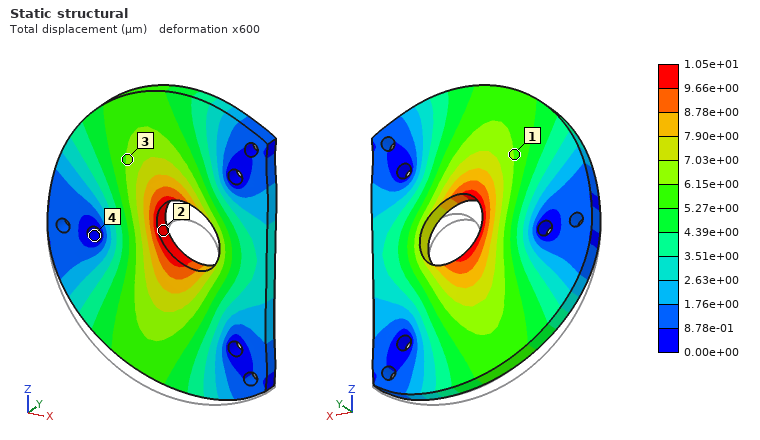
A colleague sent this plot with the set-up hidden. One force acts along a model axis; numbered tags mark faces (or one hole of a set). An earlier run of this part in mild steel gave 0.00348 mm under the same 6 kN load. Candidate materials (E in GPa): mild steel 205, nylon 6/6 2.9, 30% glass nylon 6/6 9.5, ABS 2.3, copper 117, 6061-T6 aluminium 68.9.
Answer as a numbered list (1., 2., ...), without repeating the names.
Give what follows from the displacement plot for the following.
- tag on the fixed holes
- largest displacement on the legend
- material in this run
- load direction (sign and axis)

1. 4
2. 1.05e+01 µm
3. 6061-T6 aluminium
4. +Z
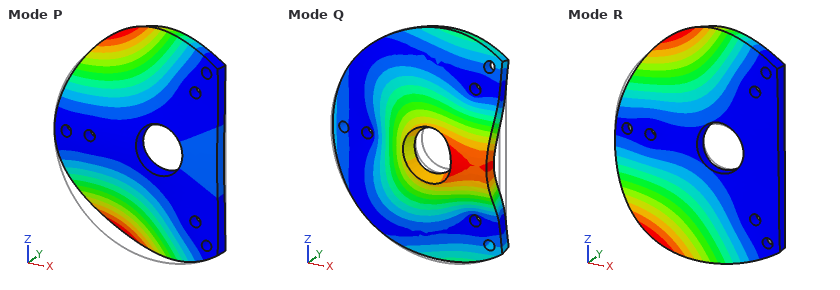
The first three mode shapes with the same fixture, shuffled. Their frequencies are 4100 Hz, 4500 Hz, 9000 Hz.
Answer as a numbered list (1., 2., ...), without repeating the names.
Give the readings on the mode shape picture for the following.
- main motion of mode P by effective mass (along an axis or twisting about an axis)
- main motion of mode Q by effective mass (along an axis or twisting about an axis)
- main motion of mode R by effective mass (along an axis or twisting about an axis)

1. along Y
2. along Y
3. twisting about X
